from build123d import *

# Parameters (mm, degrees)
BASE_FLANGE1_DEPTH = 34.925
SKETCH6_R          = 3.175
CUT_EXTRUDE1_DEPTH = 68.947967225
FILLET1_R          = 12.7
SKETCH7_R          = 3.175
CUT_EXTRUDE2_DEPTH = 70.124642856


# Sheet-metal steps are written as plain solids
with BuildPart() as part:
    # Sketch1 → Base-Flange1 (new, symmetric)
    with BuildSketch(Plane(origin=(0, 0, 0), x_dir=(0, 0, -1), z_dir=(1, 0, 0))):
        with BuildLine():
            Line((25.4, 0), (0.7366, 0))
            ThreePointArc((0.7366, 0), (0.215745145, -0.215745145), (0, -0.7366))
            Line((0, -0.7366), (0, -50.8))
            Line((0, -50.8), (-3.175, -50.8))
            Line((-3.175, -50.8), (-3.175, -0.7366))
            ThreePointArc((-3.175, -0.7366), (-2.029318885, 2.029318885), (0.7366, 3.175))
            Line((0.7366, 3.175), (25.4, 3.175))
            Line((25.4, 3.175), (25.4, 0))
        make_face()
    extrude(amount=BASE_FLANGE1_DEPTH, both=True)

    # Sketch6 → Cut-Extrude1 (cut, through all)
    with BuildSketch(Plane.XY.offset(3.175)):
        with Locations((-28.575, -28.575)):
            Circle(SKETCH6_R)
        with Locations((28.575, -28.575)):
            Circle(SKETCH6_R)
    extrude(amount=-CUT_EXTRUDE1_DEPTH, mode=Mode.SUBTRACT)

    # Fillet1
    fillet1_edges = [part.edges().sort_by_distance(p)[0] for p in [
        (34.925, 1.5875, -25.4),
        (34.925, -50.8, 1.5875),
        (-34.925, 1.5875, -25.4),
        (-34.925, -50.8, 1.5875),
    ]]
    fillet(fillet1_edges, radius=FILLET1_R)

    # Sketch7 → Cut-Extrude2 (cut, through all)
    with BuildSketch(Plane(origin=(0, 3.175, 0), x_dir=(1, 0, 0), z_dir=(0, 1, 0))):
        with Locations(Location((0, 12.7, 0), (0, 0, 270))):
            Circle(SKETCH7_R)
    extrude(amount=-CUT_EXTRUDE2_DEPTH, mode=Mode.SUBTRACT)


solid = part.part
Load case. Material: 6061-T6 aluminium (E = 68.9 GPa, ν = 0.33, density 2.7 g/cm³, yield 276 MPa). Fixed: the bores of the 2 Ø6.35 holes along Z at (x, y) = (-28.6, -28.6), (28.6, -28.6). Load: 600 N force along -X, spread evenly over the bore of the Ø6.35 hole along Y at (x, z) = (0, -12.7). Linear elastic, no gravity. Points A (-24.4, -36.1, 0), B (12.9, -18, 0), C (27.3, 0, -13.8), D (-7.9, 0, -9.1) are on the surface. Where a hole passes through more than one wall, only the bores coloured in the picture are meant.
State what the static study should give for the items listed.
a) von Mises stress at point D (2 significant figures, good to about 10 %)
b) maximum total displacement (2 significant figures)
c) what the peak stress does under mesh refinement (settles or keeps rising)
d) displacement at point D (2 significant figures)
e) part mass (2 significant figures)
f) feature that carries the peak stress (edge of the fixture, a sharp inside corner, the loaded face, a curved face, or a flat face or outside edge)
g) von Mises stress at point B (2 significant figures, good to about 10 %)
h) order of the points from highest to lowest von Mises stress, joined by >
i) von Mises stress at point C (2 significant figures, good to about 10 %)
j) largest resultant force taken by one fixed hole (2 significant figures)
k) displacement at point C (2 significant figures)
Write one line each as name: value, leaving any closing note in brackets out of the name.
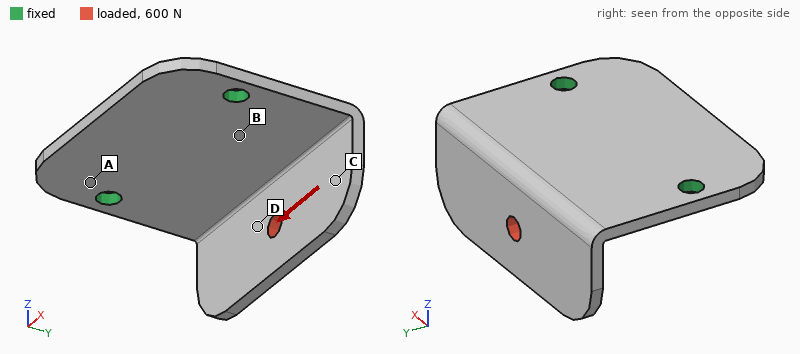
von Mises stress at point D: 22 MPa
maximum total displacement: 0.18 mm
what the peak stress does under mesh refinement: keeps rising
displacement at point D: 0.062 mm
part mass: 45 g
feature that carries the peak stress: edge of the fixture
von Mises stress at point B: 27 MPa
order of the points from highest to lowest von Mises stress, joined by >: B > D > C > A
von Mises stress at point C: 14 MPa
largest resultant force taken by one fixed hole: 450 N
displacement at point C: 0.14 mm
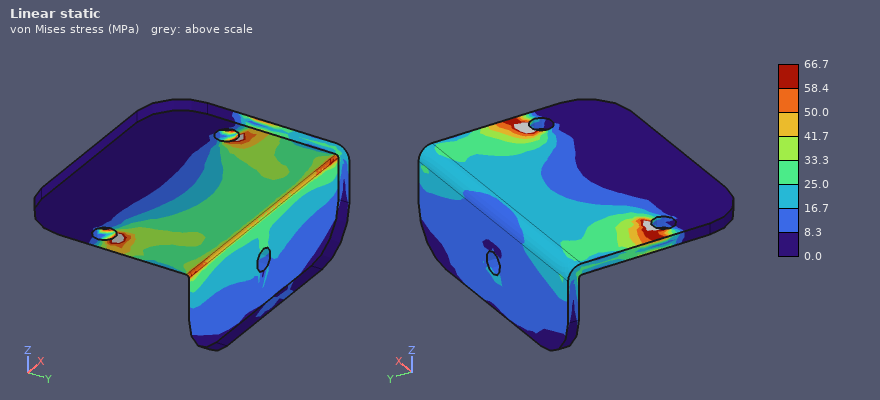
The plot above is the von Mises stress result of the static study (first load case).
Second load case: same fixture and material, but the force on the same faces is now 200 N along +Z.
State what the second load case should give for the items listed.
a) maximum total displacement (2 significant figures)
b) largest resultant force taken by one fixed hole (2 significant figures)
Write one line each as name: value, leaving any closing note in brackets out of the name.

maximum total displacement: 0.26 mm
largest resultant force taken by one fixed hole: 100 N
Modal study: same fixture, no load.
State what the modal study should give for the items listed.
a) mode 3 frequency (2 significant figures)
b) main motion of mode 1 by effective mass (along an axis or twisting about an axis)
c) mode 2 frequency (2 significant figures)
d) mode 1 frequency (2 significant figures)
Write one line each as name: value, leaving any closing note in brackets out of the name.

mode 3 frequency: 3000 Hz
main motion of mode 1 by effective mass: along Z
mode 2 frequency: 2000 Hz
mode 1 frequency: 1100 Hz
